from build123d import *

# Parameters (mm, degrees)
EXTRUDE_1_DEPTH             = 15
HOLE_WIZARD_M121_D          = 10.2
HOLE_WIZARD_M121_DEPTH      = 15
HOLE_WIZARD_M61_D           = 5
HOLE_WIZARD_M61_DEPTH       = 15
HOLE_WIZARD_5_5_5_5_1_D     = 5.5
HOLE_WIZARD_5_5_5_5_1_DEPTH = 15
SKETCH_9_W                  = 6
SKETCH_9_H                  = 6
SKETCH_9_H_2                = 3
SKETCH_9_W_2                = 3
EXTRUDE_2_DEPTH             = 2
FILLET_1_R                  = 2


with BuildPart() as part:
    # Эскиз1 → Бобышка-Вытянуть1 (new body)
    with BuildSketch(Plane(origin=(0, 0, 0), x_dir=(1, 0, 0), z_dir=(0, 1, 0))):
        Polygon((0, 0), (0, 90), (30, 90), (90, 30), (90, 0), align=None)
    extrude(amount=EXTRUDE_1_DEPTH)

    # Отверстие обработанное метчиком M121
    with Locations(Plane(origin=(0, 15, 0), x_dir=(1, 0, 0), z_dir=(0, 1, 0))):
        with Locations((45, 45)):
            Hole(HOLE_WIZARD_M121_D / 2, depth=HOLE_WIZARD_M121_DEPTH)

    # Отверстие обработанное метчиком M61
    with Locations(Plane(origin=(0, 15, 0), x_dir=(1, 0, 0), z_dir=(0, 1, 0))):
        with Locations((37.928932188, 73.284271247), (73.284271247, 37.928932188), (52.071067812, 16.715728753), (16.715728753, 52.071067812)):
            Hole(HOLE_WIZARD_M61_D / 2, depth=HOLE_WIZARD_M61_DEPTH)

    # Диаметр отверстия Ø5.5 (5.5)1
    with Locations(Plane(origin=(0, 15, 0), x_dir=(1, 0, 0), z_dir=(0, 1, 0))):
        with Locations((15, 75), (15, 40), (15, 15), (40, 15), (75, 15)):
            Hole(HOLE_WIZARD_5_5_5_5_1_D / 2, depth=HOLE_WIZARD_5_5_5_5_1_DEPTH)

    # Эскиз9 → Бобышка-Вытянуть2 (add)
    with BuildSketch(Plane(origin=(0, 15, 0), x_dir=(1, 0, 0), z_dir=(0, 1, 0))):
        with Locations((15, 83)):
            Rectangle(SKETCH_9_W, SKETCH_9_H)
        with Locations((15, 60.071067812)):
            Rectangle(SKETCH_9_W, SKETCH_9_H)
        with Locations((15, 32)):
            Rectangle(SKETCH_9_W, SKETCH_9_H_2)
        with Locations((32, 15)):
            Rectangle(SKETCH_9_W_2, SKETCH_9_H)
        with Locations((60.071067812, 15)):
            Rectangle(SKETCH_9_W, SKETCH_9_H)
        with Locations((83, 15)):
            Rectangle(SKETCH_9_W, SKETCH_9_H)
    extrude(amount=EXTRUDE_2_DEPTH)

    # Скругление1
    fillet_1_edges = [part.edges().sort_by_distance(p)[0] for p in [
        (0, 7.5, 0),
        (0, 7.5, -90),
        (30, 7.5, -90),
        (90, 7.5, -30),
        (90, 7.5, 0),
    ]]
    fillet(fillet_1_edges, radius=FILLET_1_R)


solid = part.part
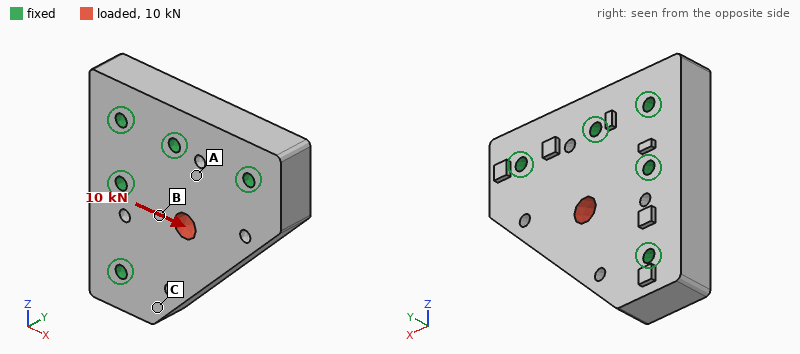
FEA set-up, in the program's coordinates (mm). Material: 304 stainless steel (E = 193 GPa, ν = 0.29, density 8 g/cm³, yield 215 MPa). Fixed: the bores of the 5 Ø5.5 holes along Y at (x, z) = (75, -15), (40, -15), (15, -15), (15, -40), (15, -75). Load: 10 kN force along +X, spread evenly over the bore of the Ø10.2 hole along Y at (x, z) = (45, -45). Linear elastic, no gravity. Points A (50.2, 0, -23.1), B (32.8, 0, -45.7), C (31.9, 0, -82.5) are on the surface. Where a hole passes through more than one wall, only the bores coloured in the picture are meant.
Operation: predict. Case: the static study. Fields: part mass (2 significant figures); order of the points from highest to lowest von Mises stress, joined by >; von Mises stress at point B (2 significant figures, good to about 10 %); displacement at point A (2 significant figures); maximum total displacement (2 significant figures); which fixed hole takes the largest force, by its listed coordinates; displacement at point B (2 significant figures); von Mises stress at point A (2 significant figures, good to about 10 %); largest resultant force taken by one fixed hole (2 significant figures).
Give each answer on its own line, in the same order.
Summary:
730 g
B > A > C
18 MPa
0.51 µm
3.1 µm
(15, -40)
1.6 µm
7.8 MPa
4.0 kN
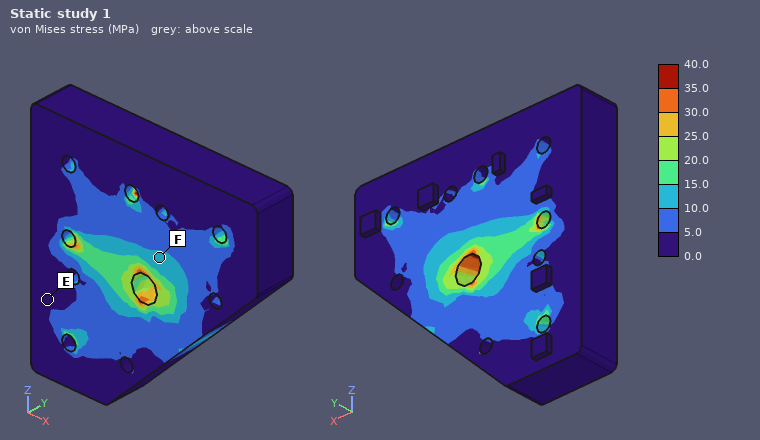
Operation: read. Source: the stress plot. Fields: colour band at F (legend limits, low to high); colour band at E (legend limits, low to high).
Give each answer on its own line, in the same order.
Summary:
10.0 to 15.0 MPa
0.0 to 5.0 MPa
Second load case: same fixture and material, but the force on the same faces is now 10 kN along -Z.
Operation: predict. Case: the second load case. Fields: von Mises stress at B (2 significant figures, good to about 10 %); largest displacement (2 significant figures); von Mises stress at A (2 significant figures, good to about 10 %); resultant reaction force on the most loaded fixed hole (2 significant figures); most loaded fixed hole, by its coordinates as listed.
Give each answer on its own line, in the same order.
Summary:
11 MPa
3.1 µm
8.8 MPa
4.0 kN
(40, -15)
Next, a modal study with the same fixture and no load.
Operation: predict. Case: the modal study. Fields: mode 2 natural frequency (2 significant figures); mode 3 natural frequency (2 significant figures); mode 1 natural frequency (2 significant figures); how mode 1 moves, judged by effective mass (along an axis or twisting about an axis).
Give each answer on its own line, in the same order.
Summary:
17 kHz
23 kHz
9100 Hz
along Y
